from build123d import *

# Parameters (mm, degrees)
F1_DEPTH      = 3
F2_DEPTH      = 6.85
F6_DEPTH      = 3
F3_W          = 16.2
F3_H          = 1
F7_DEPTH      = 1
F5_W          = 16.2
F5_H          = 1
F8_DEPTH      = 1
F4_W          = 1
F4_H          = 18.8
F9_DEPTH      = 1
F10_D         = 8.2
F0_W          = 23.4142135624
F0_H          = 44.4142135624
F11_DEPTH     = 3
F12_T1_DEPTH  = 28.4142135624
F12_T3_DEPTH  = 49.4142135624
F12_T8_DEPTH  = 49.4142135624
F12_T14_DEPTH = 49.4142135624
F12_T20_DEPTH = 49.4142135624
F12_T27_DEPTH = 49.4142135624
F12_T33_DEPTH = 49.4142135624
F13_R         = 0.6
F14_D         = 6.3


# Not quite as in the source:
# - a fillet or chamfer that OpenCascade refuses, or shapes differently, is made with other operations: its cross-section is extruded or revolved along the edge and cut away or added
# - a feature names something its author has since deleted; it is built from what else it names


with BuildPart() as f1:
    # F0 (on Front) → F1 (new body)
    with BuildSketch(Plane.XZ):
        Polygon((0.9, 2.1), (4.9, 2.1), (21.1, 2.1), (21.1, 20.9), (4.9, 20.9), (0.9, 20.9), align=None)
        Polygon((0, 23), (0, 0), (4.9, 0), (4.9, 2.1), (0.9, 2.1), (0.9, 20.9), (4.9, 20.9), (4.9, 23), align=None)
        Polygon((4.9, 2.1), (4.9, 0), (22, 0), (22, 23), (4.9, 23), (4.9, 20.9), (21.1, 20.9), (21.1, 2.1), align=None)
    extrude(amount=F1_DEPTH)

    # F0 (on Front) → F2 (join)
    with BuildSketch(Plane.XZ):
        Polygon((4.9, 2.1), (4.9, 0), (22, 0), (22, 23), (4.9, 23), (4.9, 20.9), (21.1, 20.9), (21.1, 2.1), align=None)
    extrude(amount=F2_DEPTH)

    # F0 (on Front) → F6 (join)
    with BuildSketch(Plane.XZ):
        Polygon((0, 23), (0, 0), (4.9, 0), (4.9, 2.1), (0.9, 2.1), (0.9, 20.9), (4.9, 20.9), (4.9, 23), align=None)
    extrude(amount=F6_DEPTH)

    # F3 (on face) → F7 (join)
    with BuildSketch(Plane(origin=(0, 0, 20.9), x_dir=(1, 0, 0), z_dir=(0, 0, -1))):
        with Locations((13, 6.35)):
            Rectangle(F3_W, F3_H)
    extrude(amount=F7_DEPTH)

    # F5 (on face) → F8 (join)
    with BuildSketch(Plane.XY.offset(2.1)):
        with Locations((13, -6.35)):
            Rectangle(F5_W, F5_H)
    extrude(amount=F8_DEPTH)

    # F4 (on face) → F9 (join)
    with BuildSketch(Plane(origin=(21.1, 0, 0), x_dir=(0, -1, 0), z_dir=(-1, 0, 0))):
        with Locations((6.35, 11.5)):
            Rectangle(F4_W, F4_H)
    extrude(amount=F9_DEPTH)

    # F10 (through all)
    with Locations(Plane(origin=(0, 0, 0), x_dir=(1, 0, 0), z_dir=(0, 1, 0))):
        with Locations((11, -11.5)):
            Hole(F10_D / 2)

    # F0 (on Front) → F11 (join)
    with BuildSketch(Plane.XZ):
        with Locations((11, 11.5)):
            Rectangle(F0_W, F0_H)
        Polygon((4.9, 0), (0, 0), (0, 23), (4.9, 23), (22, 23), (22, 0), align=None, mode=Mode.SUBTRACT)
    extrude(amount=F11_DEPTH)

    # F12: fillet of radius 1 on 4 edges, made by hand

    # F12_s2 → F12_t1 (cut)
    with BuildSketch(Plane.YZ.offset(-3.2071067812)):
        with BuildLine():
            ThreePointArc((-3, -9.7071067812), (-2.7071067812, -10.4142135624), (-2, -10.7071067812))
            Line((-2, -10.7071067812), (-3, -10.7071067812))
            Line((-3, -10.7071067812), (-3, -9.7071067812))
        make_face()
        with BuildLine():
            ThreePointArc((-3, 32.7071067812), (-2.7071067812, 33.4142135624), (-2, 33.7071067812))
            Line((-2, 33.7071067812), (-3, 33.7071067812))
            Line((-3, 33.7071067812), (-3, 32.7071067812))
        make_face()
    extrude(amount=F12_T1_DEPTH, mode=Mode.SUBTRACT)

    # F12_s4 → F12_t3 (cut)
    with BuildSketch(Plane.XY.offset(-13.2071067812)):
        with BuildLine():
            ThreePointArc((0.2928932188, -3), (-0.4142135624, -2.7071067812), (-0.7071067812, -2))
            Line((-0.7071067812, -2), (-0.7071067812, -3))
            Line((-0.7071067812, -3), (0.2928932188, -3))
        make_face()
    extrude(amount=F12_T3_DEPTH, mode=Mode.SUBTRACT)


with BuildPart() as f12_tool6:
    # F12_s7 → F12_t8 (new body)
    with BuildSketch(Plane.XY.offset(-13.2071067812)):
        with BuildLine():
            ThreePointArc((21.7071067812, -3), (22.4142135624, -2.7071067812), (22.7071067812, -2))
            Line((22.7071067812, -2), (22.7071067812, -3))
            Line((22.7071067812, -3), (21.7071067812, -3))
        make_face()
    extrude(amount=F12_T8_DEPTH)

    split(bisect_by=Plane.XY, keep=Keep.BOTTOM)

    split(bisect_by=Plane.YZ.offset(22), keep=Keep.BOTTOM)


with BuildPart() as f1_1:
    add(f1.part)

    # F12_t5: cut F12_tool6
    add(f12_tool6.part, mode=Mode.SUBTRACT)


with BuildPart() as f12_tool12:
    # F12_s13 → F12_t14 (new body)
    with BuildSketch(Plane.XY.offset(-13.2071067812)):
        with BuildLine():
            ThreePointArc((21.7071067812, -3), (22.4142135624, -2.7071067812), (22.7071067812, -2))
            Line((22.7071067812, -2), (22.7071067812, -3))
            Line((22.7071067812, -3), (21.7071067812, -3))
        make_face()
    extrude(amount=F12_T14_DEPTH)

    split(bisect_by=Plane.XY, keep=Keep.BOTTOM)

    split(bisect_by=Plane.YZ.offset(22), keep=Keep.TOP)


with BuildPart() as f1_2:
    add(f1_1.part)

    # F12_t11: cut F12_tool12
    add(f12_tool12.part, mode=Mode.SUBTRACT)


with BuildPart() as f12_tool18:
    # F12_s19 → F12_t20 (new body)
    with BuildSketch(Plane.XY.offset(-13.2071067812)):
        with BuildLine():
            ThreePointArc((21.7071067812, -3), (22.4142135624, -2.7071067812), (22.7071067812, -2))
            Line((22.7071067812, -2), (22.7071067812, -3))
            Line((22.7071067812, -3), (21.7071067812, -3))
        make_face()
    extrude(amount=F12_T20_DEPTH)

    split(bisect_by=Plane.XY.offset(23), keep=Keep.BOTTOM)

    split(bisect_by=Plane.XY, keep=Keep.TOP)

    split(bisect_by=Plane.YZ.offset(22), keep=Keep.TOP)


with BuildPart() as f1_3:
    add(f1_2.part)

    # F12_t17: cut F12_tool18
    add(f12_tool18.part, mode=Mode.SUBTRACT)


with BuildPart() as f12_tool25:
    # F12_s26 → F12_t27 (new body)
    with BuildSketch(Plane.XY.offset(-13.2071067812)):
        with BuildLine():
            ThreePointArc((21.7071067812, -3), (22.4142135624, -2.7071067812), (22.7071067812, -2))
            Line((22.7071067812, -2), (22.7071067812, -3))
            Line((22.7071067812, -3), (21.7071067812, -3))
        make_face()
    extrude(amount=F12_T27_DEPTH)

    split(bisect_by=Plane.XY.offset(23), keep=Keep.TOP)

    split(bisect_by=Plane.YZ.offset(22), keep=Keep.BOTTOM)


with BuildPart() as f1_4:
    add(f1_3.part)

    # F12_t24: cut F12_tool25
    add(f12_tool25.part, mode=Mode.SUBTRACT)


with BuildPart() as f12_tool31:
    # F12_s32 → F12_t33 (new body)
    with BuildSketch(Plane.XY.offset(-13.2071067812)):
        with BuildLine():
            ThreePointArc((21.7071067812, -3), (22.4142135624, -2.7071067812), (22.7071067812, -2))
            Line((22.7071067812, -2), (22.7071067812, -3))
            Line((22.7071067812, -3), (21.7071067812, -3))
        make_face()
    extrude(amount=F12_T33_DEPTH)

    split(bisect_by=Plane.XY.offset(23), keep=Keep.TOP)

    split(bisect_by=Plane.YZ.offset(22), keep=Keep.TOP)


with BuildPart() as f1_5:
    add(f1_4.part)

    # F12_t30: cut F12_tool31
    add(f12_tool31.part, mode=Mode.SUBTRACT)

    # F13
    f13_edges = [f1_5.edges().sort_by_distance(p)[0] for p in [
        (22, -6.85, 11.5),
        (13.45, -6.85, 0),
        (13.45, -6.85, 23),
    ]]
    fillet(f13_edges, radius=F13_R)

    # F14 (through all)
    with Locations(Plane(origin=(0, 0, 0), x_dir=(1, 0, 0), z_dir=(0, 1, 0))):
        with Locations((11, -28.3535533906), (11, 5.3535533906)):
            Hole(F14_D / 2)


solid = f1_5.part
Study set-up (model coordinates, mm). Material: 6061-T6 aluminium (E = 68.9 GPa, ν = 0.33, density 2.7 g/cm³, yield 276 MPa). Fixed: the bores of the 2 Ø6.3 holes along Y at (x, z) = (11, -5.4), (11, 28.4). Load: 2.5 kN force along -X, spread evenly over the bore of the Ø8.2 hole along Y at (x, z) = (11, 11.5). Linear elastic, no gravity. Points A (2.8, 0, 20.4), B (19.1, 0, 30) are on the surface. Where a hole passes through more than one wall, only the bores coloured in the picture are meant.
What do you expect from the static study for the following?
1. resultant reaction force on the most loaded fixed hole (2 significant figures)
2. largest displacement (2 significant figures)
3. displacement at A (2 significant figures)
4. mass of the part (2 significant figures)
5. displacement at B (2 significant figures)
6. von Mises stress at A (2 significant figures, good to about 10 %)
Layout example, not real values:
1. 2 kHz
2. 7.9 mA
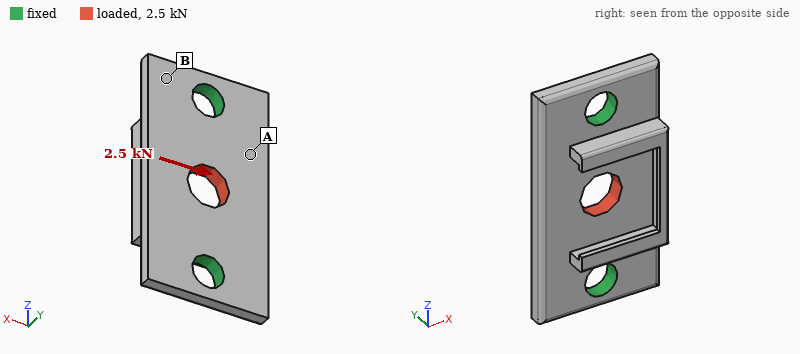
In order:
1. 1.3 kN
2. 16 µm
3. 8.2 µm
4. 8.5 g
5. 2.9 µm
6. 27 MPa
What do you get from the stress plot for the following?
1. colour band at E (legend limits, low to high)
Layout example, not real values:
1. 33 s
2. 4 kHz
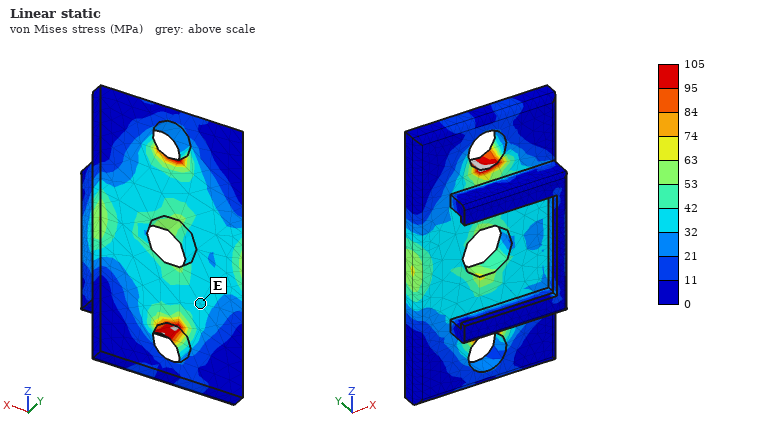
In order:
1. 32 to 42 MPa
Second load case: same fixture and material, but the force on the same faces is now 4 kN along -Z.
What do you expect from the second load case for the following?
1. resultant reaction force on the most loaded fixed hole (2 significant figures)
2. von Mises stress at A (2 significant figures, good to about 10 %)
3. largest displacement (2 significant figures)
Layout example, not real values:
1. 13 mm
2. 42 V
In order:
1. 2.0 kN
2. 17 MPa
3. 10 µm
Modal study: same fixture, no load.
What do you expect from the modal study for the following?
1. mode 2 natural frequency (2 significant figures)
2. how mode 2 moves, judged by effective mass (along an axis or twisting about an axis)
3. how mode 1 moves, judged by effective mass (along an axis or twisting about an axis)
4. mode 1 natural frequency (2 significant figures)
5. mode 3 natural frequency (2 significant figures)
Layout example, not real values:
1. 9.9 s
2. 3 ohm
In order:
1. 15 kHz
2. along Y
3. twisting about Z
4. 14 kHz
5. 25 kHz
